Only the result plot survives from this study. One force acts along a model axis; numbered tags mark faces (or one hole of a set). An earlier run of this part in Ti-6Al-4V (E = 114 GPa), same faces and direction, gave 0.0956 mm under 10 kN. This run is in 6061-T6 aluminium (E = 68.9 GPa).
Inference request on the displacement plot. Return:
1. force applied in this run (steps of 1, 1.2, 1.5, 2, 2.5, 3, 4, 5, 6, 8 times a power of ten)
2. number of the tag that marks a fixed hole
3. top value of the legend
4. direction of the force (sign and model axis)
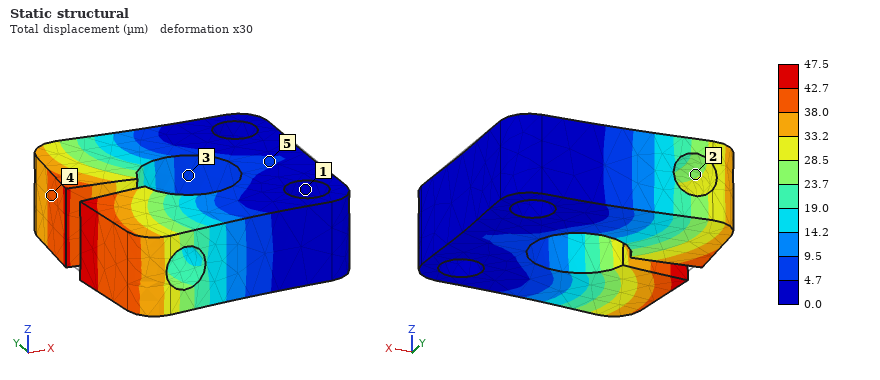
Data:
3 kN
1
47.5 µm
-X
